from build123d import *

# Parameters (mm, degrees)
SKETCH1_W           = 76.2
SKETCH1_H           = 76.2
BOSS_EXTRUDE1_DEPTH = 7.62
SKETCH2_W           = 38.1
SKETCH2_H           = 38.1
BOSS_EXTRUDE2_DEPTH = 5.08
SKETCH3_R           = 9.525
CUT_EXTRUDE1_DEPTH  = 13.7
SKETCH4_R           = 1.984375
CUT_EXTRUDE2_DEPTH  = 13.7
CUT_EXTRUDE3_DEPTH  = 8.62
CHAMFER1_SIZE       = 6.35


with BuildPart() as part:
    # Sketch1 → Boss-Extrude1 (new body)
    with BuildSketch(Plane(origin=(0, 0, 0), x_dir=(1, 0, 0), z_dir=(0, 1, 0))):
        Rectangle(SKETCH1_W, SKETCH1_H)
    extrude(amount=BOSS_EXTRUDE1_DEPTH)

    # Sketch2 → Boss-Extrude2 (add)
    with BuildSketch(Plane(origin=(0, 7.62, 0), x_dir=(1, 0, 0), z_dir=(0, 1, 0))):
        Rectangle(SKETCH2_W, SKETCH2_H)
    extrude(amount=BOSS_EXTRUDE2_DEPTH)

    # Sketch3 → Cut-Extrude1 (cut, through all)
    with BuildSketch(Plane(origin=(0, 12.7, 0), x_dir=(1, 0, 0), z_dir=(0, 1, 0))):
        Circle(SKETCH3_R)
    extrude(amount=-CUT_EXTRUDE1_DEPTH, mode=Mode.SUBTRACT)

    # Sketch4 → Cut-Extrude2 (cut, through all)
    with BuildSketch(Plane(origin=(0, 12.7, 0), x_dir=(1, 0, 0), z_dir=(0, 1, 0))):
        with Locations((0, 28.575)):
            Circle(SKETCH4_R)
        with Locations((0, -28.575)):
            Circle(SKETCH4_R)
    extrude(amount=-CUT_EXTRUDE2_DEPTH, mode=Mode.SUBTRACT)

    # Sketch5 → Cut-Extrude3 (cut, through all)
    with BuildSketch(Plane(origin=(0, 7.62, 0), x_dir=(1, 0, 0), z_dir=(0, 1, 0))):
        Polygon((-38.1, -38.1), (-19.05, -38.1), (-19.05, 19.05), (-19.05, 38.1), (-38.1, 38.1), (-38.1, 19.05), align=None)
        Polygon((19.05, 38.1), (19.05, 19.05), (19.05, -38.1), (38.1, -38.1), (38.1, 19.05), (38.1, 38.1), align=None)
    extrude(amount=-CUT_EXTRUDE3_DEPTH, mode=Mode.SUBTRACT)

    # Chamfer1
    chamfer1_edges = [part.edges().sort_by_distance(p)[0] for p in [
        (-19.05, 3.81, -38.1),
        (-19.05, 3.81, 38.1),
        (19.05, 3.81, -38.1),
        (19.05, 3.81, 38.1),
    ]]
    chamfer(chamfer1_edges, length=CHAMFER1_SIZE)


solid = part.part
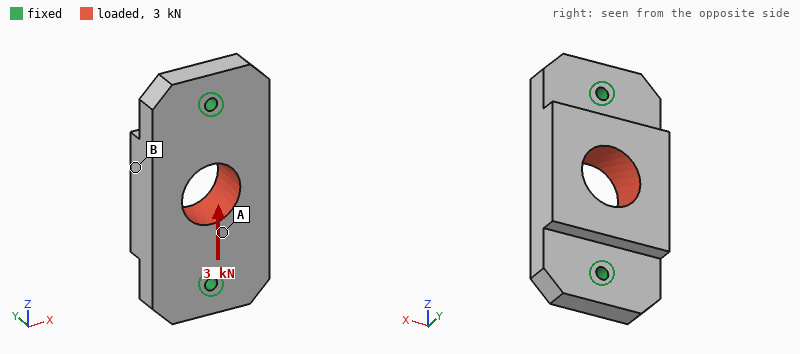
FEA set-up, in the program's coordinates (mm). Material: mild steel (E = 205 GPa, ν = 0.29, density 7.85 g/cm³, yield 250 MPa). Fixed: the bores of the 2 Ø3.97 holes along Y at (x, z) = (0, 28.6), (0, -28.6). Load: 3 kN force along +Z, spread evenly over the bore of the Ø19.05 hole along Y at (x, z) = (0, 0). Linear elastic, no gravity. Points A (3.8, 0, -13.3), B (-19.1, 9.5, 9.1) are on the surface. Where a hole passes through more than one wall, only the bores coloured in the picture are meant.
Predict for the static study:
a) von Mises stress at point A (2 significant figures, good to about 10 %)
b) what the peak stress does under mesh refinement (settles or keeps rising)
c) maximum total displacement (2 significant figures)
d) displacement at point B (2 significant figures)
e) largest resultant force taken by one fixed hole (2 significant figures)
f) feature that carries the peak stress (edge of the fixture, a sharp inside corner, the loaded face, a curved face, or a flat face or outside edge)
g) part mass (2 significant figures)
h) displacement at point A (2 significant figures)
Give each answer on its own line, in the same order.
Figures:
6.9 MPa
keeps rising
1.2 µm
0.90 µm
1.5 kN
edge of the fixture
200 g
0.71 µm
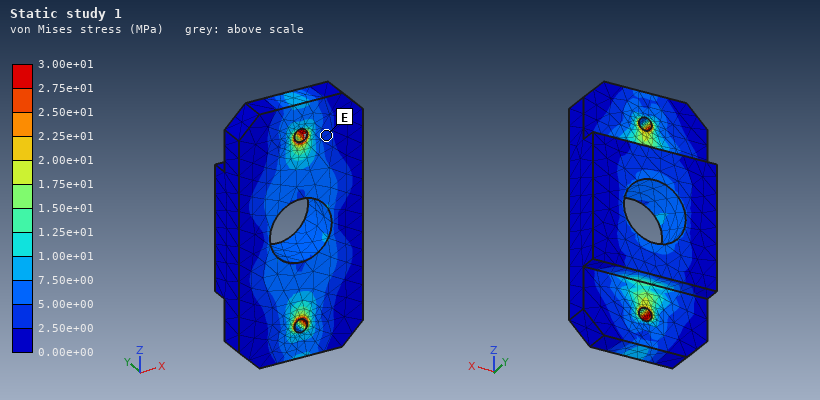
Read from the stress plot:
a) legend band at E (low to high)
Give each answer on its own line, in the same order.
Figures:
2.50e+00 to 5.00e+00 MPa
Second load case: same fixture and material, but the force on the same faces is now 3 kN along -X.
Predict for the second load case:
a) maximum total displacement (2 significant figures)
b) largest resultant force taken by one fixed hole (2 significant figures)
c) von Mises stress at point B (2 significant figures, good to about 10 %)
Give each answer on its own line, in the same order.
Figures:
5.6 µm
1.5 kN
7.6 MPa
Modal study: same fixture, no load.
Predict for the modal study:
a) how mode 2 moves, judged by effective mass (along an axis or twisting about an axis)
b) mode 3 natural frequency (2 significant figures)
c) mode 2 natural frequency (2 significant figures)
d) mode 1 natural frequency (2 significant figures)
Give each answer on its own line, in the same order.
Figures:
along Y
16 kHz
9200 Hz
7000 Hz
